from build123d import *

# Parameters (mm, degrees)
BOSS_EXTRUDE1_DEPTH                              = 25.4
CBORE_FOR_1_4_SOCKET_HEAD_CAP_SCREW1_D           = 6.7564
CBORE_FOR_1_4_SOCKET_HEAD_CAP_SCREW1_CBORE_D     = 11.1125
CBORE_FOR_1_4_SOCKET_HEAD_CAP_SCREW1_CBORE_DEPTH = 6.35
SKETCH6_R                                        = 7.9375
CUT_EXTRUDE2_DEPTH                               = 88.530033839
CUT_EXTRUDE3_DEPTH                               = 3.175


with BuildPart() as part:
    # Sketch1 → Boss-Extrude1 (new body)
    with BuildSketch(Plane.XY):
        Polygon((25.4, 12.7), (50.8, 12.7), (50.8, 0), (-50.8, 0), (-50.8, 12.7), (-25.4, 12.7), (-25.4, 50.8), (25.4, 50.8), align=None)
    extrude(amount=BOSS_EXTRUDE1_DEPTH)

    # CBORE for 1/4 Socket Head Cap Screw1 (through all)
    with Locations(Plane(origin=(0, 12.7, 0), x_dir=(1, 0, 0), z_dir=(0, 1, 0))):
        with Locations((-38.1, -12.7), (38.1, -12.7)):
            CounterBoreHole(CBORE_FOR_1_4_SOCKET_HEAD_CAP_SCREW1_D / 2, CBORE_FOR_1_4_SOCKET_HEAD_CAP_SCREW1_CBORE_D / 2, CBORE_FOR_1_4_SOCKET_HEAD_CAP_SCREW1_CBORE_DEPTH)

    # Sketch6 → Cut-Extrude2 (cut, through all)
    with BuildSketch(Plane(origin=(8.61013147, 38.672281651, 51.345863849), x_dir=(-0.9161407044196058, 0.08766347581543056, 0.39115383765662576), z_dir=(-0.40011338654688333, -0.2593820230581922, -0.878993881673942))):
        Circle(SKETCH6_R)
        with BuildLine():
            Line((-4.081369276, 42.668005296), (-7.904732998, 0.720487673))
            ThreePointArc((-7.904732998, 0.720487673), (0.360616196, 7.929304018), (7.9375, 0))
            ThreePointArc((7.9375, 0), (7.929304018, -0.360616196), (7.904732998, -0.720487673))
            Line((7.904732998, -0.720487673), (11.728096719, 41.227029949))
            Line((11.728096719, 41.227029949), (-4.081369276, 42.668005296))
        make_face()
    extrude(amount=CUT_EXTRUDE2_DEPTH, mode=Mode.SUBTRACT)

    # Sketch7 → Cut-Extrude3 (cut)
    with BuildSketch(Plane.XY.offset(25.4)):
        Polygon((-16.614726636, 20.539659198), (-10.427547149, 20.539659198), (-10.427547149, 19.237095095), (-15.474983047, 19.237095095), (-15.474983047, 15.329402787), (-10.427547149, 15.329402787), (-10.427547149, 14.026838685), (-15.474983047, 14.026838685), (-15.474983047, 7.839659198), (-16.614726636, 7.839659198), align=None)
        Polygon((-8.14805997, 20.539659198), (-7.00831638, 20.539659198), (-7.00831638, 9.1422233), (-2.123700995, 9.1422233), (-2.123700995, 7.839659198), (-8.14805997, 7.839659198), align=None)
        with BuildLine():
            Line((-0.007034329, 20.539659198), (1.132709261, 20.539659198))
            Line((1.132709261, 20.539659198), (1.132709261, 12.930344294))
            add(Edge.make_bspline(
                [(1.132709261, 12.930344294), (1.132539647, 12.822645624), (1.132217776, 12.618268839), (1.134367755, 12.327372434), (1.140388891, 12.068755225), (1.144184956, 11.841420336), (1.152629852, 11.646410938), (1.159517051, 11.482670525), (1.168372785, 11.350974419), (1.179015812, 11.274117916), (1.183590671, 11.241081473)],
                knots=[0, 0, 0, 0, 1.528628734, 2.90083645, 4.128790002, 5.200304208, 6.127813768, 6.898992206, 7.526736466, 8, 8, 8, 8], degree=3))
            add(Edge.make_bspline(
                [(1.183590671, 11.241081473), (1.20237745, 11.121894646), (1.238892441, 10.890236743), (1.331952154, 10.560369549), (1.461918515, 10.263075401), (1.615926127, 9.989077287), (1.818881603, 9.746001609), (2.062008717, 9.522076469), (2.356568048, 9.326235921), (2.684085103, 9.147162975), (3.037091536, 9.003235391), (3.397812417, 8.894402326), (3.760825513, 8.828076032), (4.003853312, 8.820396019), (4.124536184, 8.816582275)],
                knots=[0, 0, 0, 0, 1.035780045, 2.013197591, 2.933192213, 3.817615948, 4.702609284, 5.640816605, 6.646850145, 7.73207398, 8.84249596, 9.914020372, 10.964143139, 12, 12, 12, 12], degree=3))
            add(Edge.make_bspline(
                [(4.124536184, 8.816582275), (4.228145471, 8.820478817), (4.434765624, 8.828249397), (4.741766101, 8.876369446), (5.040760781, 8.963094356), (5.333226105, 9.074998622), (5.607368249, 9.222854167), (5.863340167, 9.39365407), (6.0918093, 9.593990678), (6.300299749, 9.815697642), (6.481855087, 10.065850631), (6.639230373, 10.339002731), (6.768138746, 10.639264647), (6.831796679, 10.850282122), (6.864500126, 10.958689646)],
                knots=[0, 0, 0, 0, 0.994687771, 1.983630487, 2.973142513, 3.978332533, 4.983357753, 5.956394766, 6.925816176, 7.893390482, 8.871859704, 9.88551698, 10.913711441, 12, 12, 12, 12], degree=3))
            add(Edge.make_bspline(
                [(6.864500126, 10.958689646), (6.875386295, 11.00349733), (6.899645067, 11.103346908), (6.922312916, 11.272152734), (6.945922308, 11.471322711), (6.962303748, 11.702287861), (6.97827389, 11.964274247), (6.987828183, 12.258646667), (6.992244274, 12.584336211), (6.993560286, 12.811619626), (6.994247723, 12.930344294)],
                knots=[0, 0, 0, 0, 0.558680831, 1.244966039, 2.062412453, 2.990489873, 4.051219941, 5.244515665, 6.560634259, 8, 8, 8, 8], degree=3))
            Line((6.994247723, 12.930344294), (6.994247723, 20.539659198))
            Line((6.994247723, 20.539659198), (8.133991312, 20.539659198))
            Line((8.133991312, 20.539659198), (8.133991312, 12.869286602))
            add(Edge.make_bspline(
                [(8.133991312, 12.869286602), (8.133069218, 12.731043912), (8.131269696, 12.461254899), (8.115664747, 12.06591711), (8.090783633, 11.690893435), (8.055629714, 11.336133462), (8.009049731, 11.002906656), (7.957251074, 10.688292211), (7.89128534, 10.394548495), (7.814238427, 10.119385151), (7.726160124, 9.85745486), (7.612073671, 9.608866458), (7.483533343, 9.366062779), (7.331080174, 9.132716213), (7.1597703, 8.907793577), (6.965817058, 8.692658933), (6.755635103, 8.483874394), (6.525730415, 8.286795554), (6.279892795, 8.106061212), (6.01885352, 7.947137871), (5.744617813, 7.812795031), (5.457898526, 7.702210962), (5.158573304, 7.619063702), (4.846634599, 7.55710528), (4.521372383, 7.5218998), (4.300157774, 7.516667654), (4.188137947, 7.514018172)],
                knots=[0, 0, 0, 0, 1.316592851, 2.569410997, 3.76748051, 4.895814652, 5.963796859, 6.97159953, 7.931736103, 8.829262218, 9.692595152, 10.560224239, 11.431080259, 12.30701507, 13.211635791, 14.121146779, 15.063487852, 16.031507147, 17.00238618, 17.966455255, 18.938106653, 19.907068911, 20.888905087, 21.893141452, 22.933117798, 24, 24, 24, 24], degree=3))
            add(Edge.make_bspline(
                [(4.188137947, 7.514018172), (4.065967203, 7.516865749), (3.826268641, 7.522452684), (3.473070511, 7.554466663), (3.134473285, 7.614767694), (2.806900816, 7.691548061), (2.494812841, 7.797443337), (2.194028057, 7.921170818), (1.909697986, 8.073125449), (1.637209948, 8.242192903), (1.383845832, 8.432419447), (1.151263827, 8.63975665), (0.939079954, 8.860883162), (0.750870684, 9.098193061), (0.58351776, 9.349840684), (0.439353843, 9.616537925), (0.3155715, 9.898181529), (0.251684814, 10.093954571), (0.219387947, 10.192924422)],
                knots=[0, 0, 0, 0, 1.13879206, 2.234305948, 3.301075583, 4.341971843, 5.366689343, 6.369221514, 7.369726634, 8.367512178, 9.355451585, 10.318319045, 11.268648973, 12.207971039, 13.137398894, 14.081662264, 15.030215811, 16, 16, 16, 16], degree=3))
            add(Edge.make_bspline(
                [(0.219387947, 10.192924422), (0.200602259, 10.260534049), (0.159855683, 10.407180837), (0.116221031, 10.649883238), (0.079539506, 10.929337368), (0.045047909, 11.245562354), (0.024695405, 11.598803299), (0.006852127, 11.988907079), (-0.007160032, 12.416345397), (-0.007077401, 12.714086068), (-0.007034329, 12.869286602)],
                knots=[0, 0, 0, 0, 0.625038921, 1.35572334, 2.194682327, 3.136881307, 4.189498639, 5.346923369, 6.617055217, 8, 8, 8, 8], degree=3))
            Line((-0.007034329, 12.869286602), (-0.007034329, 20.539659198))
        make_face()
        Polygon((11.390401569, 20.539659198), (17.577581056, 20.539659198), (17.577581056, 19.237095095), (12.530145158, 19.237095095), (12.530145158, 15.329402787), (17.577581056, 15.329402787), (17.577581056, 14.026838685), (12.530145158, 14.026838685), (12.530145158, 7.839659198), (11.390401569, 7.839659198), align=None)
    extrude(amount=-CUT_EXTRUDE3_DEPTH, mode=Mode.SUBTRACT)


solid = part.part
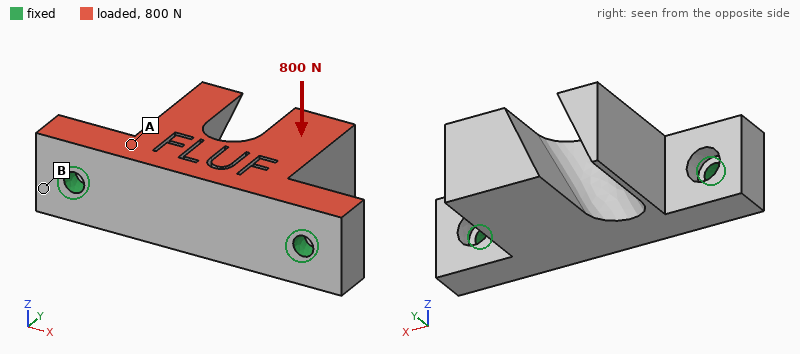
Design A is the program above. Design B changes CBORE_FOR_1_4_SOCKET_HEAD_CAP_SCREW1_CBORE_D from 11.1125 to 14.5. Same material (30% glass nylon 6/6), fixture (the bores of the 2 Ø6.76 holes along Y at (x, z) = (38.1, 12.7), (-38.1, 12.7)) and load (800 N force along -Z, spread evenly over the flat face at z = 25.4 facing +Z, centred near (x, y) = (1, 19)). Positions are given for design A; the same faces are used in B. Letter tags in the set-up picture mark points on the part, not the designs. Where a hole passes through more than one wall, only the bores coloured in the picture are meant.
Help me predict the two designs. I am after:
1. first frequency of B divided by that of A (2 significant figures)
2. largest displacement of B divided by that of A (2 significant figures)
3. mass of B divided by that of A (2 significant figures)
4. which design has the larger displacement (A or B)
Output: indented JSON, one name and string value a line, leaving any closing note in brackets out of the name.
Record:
{
  "first frequency of B divided by that of A": "0.96",
  "largest displacement of B divided by that of A": "1.1",
  "mass of B divided by that of A": "0.99",
  "which design has the larger displacement": "B"
}
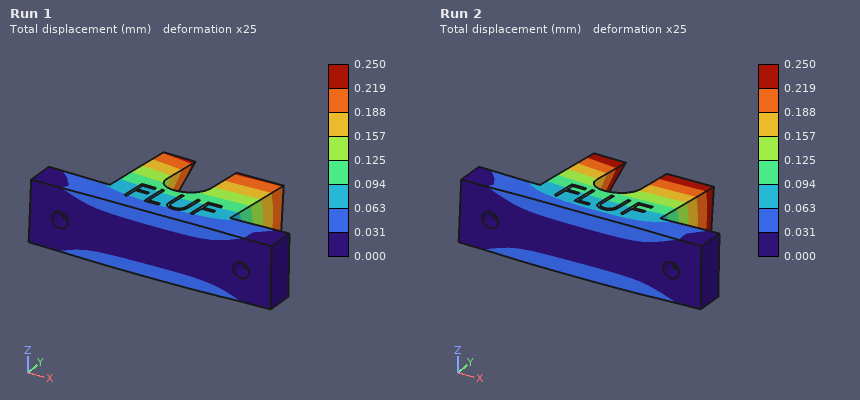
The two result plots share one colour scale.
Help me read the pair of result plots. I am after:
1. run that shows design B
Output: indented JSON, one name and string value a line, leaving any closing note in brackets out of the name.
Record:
{
  "run that shows design B": "Run 2"
}
